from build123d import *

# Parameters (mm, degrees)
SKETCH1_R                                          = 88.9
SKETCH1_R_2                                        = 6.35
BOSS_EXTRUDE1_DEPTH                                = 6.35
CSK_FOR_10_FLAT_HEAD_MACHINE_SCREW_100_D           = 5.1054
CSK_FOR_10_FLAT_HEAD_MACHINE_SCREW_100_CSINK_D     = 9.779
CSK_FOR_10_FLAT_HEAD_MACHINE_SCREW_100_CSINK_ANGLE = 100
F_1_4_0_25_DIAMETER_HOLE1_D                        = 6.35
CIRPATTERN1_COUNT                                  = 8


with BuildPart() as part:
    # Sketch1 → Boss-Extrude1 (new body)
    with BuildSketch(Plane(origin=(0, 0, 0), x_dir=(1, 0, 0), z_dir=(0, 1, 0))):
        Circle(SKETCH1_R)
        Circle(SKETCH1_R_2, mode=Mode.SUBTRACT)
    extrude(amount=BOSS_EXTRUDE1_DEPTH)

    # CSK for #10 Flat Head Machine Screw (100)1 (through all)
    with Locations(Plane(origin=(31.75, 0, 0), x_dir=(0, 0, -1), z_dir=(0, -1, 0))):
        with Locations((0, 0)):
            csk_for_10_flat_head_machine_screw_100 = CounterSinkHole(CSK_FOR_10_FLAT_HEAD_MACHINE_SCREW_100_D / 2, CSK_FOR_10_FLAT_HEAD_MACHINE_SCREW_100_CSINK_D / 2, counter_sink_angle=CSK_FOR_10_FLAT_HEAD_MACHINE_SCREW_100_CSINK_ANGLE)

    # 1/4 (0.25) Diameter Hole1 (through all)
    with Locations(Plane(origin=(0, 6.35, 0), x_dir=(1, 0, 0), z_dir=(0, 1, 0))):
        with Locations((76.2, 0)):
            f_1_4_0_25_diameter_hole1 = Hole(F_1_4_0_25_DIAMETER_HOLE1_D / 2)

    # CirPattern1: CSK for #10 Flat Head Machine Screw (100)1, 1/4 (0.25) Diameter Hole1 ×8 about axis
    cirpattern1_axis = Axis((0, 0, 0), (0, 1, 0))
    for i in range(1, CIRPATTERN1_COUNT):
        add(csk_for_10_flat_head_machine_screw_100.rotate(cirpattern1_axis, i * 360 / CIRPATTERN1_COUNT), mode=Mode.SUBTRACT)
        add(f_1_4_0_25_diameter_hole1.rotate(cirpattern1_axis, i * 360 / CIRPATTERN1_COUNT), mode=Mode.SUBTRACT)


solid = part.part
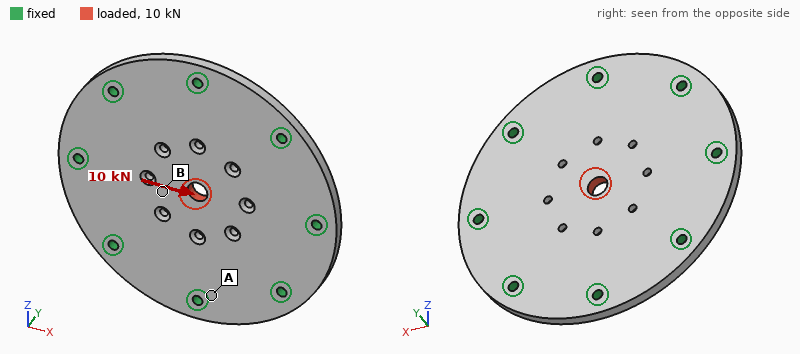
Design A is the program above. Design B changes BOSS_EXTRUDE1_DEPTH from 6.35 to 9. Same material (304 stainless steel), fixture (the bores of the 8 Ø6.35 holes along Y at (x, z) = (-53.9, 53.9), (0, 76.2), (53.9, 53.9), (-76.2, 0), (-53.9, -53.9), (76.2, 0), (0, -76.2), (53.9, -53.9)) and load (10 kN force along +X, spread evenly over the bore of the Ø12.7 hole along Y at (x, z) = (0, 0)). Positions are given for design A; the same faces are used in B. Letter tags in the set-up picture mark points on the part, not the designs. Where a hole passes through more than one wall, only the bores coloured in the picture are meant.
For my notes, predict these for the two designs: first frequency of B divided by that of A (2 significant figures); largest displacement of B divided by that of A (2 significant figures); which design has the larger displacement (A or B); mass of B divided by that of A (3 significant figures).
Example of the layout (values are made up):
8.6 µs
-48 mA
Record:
1.4
0.71
A
1.42
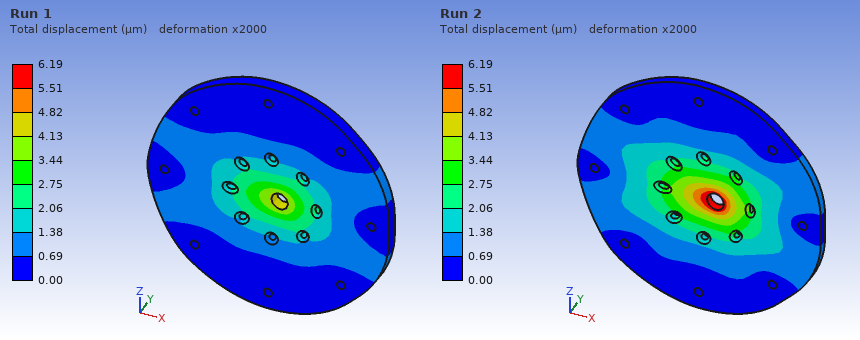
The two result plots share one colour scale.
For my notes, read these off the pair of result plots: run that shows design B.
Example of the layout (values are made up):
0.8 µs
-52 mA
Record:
Run 1
